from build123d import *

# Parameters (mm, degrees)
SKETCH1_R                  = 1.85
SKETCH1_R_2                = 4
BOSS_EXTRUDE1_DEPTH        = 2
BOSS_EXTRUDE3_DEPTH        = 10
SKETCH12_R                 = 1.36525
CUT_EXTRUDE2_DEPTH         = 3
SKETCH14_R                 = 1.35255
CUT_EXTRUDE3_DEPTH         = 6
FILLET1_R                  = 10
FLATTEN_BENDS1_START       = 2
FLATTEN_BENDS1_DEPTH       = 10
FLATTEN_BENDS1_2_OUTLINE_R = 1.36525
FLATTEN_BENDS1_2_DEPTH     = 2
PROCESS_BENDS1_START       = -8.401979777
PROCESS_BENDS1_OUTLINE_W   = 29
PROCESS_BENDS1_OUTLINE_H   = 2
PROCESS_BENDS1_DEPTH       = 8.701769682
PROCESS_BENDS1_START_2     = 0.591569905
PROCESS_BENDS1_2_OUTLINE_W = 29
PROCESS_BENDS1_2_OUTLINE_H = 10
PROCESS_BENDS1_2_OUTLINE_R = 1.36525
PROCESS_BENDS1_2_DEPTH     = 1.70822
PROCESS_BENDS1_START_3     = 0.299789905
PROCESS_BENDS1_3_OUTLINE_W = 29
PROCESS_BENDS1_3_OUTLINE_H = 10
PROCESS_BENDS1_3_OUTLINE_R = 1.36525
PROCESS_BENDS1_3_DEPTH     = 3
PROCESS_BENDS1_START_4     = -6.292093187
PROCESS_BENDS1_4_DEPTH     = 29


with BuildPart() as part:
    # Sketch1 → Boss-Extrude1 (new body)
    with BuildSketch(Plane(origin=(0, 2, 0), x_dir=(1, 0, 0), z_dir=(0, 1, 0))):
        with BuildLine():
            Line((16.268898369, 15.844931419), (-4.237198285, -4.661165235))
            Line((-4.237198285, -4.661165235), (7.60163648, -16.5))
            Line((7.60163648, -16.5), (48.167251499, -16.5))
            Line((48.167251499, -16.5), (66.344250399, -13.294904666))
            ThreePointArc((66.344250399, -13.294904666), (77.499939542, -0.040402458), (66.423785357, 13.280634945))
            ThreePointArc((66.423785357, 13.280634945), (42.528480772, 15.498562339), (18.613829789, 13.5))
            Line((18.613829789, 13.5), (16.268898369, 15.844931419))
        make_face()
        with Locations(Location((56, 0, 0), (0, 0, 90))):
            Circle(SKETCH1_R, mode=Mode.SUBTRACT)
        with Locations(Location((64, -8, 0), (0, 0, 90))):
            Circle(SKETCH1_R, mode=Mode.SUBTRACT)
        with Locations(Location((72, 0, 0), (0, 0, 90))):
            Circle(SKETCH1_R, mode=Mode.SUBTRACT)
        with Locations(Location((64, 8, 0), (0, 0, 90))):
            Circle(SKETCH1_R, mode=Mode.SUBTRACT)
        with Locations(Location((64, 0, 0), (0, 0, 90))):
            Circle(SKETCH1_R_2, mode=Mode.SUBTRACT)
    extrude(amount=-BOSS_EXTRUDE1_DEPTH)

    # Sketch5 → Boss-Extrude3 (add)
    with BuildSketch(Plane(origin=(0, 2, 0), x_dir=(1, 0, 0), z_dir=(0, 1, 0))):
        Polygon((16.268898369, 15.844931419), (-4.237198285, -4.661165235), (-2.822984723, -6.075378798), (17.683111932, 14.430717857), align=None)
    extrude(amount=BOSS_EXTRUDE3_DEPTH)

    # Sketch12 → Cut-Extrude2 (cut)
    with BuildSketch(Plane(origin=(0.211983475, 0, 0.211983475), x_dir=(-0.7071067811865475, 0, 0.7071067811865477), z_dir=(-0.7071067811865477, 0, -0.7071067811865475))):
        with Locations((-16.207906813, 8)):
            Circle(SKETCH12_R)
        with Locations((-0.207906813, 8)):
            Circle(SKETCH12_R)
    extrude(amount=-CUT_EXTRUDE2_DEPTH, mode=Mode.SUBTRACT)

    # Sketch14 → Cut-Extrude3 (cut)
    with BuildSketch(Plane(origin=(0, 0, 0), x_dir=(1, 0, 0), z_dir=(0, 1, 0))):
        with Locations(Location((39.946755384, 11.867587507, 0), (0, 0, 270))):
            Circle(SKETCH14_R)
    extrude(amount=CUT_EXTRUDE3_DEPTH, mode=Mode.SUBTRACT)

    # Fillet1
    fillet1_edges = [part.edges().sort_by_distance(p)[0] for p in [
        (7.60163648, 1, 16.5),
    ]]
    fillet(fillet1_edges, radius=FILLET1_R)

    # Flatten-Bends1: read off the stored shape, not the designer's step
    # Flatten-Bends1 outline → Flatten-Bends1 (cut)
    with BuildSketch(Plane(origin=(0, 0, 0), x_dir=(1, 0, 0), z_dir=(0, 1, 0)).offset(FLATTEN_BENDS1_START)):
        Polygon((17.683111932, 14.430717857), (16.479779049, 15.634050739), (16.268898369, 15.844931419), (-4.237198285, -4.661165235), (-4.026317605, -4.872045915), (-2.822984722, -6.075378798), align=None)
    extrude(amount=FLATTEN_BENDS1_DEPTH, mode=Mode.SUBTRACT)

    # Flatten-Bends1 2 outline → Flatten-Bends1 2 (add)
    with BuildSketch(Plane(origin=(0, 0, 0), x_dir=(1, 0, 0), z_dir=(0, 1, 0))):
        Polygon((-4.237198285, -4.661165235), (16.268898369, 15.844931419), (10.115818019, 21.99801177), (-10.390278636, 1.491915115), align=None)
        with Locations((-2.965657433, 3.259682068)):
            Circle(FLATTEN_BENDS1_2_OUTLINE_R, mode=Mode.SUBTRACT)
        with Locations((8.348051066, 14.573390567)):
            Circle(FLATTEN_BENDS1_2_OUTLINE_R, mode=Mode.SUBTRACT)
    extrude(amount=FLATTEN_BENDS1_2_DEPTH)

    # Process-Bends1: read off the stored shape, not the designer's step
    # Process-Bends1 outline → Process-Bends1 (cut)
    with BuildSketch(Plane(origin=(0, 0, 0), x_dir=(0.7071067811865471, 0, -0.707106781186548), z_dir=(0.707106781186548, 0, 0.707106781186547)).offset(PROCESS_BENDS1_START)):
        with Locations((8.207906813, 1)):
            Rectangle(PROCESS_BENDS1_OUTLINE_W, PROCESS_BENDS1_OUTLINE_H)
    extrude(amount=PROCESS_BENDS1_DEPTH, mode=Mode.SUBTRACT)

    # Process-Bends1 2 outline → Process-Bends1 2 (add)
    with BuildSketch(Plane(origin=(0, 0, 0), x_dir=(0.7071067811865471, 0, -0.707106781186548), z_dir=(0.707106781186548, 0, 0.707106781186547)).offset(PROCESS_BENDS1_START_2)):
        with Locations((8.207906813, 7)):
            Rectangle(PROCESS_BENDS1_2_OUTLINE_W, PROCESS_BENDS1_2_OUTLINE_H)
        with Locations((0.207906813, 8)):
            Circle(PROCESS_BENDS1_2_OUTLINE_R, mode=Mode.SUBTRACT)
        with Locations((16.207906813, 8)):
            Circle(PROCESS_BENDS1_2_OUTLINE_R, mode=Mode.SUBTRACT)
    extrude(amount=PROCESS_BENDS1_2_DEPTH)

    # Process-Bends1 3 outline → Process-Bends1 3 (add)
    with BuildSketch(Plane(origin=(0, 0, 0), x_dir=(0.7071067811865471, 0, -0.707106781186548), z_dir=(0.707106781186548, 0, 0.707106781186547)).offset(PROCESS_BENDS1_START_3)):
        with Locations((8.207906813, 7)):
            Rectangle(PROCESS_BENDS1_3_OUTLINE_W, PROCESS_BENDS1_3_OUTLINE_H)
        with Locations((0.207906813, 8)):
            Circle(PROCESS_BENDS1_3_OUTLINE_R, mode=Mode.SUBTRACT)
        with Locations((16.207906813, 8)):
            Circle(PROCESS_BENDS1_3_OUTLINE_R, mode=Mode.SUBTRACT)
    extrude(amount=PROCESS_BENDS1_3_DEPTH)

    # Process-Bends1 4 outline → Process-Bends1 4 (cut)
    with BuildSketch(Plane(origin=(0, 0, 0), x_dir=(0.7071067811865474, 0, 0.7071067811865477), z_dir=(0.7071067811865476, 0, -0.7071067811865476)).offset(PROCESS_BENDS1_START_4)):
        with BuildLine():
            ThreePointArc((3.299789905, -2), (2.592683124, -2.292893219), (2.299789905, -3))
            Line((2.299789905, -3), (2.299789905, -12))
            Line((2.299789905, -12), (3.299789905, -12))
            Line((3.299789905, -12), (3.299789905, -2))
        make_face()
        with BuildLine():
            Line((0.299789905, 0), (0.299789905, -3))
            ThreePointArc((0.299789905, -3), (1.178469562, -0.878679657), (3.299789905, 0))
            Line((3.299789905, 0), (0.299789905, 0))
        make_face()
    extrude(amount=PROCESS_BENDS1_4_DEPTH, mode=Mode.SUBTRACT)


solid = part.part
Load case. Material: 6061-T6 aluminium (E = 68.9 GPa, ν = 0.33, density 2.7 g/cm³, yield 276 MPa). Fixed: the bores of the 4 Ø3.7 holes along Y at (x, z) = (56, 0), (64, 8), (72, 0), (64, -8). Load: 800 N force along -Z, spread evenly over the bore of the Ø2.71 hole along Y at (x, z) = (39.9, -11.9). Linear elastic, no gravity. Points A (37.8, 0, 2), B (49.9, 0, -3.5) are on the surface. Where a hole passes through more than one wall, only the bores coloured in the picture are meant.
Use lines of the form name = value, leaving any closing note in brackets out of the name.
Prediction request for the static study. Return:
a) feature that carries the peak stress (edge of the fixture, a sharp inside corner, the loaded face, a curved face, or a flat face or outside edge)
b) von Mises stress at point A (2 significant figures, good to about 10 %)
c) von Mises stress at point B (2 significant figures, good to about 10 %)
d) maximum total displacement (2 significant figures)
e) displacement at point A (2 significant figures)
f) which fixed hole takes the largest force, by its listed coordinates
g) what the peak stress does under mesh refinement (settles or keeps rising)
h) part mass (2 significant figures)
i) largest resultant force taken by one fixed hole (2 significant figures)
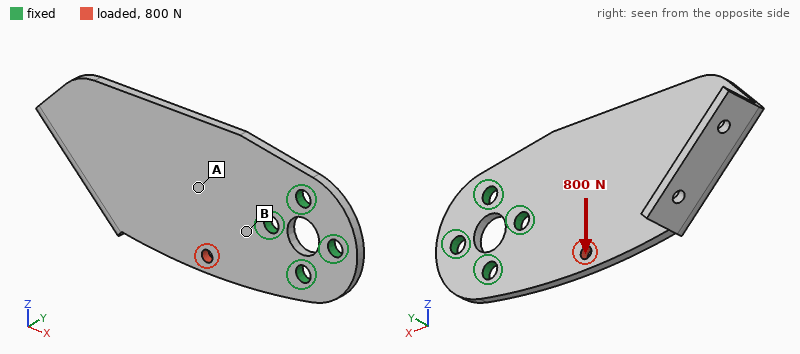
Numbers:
feature that carries the peak stress = edge of the fixture
von Mises stress at point A = 15 MPa
von Mises stress at point B = 38 MPa
maximum total displacement = 57 µm
displacement at point A = 22 µm
which fixed hole takes the largest force, by its listed coordinates = (56, 0)
what the peak stress does under mesh refinement = keeps rising
part mass = 12 g
largest resultant force taken by one fixed hole = 960 N
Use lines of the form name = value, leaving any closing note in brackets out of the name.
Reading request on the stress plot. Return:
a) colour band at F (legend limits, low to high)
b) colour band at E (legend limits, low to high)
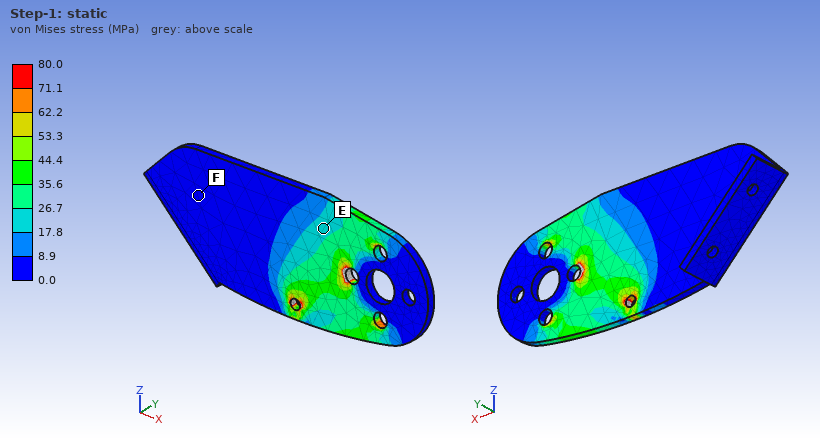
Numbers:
colour band at F = 0.0 to 8.9 MPa
colour band at E = 17.8 to 26.7 MPa
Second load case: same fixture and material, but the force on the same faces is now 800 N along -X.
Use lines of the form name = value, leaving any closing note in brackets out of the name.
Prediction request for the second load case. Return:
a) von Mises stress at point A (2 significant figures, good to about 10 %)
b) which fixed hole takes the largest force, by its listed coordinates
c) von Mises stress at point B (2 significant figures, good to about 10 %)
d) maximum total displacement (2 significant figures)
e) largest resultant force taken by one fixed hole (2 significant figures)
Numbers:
von Mises stress at point A = 7.6 MPa
which fixed hole takes the largest force, by its listed coordinates = (64, -8)
von Mises stress at point B = 21 MPa
maximum total displacement = 43 µm
largest resultant force taken by one fixed hole = 620 N
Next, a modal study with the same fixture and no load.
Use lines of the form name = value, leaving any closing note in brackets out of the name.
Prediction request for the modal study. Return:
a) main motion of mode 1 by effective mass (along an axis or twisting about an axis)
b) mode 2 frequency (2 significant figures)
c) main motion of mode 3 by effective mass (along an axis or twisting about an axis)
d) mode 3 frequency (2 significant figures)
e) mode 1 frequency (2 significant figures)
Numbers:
main motion of mode 1 by effective mass = along Y
mode 2 frequency = 1700 Hz
main motion of mode 3 by effective mass = along Y
mode 3 frequency = 2700 Hz
mode 1 frequency = 480 Hz
